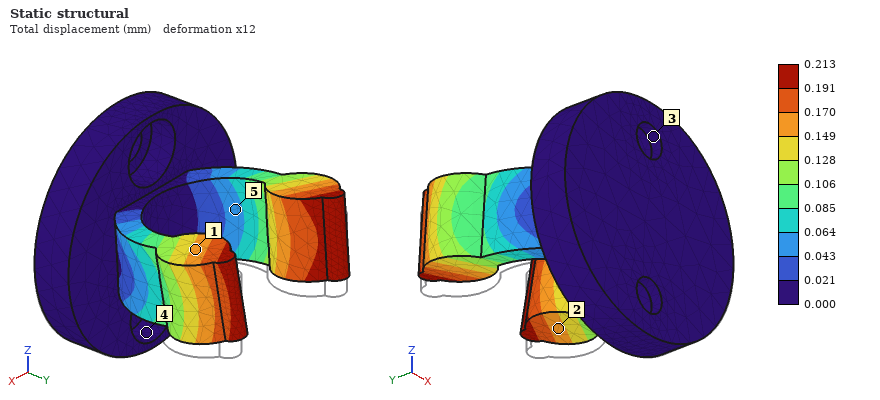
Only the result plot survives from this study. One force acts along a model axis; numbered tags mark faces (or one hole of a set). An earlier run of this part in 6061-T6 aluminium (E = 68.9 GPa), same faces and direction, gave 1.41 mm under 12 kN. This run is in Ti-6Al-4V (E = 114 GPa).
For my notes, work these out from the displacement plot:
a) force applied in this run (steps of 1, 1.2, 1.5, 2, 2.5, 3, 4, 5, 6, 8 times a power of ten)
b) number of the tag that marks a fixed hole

3 kN
3
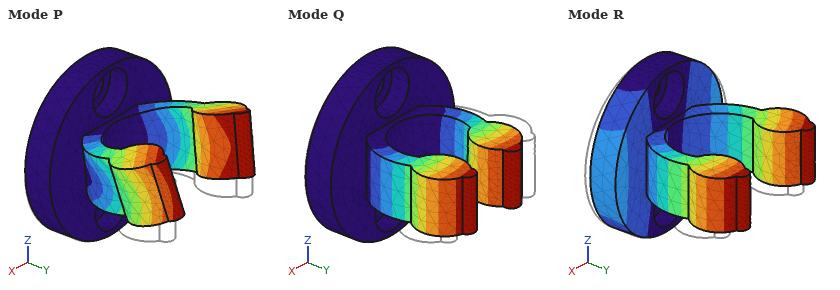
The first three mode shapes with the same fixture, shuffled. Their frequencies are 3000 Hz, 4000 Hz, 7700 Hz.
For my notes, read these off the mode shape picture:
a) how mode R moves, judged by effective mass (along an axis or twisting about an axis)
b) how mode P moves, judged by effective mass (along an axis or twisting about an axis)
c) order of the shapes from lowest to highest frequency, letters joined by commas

along X
along Z
R, Q, P
